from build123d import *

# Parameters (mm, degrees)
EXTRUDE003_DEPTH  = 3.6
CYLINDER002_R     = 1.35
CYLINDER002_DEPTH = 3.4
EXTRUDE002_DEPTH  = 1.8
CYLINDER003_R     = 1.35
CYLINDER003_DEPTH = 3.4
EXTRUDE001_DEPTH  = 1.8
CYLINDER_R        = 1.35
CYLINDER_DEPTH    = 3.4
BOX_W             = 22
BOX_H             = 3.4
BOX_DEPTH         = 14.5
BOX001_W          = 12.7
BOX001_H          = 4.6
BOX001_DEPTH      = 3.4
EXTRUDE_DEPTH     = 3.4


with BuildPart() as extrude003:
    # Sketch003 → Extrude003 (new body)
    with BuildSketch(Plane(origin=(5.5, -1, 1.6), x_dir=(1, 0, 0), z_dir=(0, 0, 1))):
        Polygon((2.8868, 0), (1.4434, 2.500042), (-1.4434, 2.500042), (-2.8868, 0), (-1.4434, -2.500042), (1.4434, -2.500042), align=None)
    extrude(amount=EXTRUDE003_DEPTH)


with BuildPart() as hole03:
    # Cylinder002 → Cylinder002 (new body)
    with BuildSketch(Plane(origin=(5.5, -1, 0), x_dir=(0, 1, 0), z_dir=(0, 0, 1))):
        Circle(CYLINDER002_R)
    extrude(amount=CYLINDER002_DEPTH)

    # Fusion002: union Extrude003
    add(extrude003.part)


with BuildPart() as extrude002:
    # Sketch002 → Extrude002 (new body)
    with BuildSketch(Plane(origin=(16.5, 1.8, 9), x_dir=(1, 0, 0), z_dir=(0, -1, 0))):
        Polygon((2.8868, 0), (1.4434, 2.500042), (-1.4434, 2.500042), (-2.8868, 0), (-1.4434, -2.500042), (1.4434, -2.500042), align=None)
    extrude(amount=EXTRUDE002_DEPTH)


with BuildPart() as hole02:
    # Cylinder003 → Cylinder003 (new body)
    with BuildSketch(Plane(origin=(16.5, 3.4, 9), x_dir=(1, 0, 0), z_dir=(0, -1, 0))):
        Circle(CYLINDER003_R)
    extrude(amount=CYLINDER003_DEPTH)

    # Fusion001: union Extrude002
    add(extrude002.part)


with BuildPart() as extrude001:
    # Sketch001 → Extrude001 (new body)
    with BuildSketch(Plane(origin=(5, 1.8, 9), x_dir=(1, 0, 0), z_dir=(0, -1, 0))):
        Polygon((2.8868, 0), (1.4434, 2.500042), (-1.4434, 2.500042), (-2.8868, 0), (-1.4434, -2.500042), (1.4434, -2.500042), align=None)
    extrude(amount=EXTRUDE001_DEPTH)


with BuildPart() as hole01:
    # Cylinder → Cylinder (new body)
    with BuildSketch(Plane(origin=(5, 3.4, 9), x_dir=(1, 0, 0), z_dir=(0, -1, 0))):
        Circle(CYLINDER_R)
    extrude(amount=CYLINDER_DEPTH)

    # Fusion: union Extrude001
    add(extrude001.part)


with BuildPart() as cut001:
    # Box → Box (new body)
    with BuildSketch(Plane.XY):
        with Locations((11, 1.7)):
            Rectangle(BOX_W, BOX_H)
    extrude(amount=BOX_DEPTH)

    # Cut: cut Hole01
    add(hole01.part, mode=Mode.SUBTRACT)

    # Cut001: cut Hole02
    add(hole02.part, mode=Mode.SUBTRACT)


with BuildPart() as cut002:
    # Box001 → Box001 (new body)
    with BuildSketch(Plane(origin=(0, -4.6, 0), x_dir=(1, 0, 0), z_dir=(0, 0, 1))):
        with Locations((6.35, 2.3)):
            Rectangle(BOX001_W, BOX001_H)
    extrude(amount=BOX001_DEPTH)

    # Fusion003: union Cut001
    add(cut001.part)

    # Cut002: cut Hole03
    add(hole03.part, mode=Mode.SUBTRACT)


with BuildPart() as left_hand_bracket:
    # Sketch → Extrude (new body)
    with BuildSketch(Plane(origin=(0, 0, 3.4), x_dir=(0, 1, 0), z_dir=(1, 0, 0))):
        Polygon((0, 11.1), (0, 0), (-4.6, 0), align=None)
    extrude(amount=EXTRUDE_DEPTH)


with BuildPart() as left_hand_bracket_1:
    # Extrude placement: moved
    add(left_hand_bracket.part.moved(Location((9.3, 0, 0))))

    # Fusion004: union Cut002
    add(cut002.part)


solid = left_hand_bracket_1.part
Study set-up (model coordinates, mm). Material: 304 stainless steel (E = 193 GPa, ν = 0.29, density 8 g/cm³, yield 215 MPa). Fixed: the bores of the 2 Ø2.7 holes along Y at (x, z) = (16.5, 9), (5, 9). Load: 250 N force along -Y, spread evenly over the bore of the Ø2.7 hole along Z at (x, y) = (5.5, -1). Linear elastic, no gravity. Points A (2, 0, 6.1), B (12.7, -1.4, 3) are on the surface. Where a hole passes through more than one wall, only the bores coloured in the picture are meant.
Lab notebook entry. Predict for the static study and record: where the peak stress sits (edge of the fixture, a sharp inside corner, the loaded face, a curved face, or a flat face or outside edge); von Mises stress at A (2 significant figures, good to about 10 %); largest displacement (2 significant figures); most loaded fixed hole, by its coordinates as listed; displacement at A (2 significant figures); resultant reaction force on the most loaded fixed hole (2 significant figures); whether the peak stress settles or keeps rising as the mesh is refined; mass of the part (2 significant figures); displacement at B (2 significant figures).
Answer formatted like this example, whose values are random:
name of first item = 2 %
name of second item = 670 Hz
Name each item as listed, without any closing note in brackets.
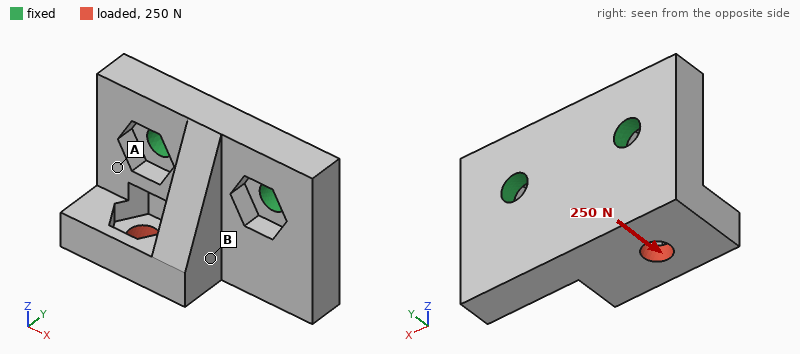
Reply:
where the peak stress sits = edge of the fixture
von Mises stress at A = 37 MPa
largest displacement = 17 µm
most loaded fixed hole, by its coordinates as listed = (5, 9)
displacement at A = 4.9 µm
resultant reaction force on the most loaded fixed hole = 230 N
whether the peak stress settles or keeps rising as the mesh is refined = keeps rising
mass of the part = 9.7 g
displacement at B = 7.0 µm
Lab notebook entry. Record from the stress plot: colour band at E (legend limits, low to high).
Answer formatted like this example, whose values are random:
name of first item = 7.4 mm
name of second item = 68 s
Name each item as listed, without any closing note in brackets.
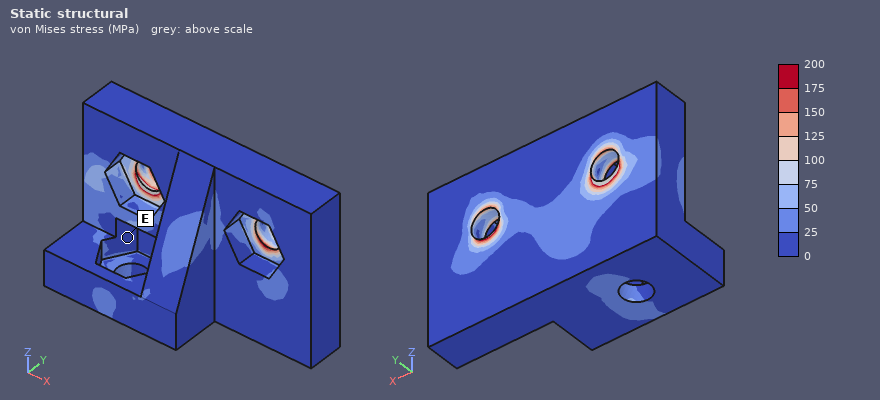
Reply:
colour band at E = 0 to 25 MPa
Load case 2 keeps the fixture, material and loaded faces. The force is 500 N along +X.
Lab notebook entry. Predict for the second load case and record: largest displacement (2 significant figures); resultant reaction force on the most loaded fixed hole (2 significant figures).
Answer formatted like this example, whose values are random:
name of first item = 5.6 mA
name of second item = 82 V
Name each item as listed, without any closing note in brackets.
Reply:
largest displacement = 5.3 µm
resultant reaction force on the most loaded fixed hole = 440 N
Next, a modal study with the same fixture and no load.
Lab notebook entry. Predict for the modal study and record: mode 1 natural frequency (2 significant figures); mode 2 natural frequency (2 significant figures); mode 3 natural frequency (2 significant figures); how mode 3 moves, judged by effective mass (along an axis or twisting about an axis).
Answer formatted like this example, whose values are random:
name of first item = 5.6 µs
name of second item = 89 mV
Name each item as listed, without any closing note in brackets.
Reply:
mode 1 natural frequency = 13 kHz
mode 2 natural frequency = 25 kHz
mode 3 natural frequency = 37 kHz
how mode 3 moves, judged by effective mass = along X
